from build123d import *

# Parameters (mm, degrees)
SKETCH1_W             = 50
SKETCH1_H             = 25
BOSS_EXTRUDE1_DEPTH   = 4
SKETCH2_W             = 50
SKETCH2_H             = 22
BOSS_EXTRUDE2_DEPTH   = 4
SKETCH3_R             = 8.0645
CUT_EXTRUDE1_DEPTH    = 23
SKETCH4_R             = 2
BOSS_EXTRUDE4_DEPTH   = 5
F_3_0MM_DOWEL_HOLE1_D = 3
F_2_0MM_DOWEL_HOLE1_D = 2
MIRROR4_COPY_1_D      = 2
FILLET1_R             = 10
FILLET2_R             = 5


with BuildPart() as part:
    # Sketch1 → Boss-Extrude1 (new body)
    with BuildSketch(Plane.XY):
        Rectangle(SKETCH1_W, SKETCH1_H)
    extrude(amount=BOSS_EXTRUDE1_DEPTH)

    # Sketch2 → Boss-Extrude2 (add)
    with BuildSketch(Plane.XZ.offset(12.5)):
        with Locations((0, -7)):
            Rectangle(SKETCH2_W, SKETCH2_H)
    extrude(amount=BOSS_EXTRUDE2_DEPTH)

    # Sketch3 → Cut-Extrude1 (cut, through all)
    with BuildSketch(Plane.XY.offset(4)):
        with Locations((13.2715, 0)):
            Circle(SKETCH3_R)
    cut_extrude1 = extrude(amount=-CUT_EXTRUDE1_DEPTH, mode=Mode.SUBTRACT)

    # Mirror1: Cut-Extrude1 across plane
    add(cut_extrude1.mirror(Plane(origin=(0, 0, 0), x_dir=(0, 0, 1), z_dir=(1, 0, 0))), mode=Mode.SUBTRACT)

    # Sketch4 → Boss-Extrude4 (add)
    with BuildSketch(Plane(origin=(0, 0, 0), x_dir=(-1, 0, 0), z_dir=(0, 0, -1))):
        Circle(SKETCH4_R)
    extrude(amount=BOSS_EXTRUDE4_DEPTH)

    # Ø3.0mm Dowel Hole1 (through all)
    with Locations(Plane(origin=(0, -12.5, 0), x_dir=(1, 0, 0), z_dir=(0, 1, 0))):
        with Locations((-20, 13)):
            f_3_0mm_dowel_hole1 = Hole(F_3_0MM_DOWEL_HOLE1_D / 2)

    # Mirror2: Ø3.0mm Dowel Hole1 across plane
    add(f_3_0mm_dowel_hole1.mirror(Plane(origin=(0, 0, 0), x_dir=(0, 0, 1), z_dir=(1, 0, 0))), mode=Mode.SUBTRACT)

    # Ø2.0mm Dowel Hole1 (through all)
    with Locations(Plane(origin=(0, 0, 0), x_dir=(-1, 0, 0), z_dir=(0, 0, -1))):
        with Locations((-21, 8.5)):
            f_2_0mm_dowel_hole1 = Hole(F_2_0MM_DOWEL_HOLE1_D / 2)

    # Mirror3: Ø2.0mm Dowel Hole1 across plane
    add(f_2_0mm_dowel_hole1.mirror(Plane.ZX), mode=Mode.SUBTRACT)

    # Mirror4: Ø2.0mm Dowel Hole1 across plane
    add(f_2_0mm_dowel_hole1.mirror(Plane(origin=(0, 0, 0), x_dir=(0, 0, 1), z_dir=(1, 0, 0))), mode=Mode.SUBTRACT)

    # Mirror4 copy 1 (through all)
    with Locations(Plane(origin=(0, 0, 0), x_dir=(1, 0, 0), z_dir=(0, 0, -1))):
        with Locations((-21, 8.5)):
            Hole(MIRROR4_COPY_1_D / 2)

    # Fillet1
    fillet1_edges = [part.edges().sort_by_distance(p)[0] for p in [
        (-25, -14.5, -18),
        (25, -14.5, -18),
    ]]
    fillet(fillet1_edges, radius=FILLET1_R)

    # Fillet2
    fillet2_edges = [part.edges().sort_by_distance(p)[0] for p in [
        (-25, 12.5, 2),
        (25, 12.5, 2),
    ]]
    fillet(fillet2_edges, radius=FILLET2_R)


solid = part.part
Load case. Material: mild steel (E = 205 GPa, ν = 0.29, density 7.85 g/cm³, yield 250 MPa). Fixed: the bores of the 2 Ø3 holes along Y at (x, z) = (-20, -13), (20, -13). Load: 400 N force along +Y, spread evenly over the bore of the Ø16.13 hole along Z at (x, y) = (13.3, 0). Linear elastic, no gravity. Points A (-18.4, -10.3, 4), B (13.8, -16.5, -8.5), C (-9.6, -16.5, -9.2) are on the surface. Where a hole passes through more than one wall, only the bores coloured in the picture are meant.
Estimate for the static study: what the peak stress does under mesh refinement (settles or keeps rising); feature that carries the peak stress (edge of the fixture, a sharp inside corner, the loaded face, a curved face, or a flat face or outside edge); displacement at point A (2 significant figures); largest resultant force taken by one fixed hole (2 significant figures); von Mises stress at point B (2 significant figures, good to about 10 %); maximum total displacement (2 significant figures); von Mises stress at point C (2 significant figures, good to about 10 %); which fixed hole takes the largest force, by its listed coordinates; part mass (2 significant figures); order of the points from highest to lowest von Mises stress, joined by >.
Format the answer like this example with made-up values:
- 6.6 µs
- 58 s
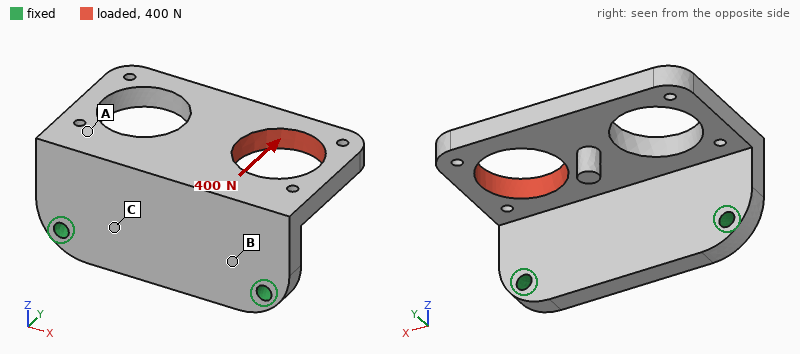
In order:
- keeps rising
- edge of the fixture
- 13 µm
- 330 N
- 37 MPa
- 47 µm
- 19 MPa
- (20, -13)
- 59 g
- B > C > A
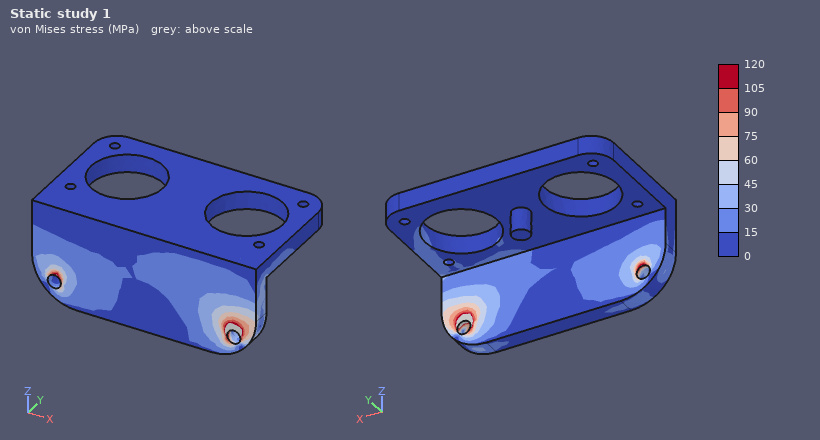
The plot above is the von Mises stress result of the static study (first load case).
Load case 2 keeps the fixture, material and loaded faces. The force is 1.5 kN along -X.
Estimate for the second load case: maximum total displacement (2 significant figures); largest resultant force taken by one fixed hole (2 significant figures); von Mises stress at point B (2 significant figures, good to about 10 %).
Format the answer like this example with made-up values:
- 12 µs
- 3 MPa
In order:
- 52 µm
- 1.1 kN
- 39 MPa
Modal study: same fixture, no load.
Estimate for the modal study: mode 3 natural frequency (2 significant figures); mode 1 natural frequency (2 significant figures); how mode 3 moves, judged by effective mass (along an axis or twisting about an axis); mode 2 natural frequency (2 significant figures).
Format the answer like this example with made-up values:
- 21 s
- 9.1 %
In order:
- 6100 Hz
- 2300 Hz
- along Y
- 4800 Hz
